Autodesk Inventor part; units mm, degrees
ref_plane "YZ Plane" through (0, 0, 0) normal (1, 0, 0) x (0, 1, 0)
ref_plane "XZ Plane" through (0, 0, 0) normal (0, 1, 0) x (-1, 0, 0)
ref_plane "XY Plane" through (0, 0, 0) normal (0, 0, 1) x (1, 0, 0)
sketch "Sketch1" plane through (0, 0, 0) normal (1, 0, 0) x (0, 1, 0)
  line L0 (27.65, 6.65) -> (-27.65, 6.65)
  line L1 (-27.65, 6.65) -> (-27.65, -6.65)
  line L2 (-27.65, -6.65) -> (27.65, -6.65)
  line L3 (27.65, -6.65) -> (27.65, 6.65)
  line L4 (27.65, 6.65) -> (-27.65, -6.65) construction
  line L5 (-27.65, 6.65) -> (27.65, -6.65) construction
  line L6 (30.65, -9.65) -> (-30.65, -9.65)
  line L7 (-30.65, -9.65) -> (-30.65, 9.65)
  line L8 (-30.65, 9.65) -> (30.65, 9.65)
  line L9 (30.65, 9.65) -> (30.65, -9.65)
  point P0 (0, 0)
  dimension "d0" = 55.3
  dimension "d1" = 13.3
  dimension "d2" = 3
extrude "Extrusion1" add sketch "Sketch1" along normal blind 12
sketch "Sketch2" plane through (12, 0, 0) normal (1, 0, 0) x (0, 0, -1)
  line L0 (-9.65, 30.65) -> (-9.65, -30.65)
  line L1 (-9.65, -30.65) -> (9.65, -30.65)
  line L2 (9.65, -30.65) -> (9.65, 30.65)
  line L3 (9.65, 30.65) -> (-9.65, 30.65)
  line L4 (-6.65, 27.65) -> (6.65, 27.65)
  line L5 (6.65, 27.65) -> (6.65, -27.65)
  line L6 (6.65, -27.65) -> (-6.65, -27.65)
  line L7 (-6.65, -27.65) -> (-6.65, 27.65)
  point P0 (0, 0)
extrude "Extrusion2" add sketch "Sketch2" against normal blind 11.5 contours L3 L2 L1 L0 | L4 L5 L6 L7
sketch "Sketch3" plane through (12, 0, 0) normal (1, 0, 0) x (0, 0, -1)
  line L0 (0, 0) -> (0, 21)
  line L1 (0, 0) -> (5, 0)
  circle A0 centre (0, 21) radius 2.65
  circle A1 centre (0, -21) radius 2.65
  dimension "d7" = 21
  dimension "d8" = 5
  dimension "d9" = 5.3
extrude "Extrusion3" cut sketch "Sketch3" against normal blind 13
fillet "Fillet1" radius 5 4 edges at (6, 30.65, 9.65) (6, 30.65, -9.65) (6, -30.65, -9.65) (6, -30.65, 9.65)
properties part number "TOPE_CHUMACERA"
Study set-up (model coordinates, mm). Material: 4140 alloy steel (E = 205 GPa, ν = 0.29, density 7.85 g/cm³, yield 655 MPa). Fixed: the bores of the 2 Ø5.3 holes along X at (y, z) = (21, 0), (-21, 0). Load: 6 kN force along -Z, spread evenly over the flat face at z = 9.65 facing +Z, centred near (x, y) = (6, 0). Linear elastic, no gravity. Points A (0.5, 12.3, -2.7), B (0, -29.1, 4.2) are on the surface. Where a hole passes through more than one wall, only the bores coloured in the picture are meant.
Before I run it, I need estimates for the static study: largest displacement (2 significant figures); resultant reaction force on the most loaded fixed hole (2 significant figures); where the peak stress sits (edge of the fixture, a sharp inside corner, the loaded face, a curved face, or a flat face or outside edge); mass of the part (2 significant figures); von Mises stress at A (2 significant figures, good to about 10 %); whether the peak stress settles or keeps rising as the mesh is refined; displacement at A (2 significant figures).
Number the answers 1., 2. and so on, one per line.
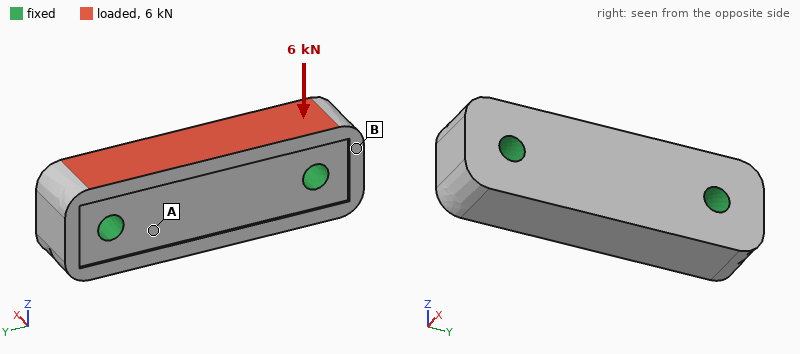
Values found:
1. 3.4 µm
2. 3.0 kN
3. edge of the fixture
4. 100 g
5. 17 MPa
6. keeps rising
7. 1.7 µm
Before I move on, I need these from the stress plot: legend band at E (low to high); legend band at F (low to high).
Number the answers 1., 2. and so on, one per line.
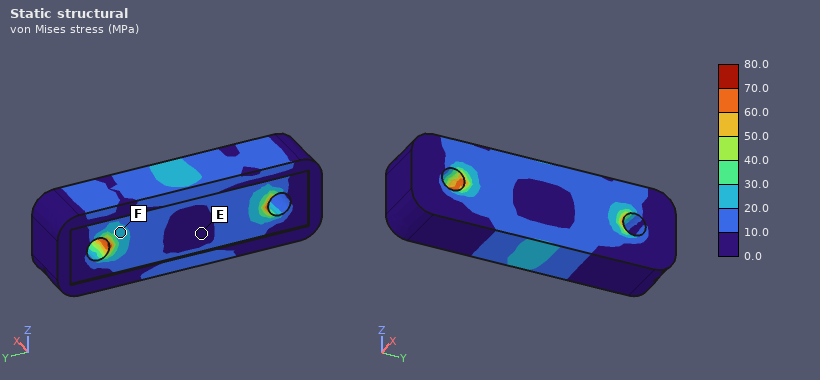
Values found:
1. 0.0 to 10.0 MPa
2. 20.0 to 30.0 MPa
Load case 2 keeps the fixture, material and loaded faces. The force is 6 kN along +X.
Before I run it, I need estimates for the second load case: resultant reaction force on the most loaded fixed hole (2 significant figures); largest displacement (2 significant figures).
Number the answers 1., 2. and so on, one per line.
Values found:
1. 3.0 kN
2. 11 µm
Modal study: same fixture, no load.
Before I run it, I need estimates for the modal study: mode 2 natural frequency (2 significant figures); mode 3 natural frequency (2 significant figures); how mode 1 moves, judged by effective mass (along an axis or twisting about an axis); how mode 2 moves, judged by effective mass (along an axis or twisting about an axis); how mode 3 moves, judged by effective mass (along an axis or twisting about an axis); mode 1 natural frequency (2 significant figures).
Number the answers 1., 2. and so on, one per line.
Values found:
1. 25 kHz
2. 30 kHz
3. along X
4. along Z
5. twisting about Y
6. 24 kHz
